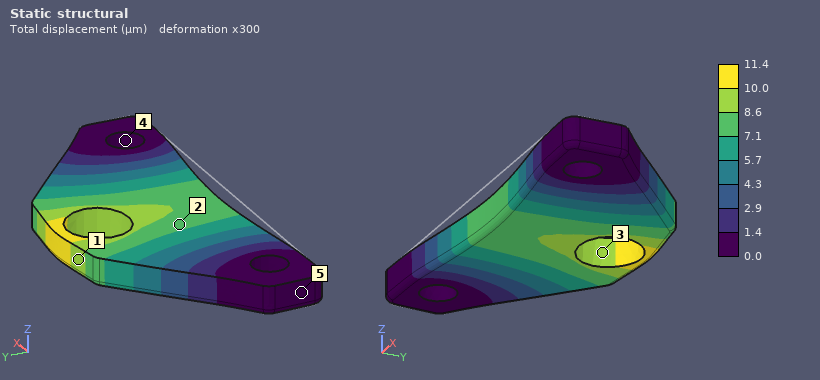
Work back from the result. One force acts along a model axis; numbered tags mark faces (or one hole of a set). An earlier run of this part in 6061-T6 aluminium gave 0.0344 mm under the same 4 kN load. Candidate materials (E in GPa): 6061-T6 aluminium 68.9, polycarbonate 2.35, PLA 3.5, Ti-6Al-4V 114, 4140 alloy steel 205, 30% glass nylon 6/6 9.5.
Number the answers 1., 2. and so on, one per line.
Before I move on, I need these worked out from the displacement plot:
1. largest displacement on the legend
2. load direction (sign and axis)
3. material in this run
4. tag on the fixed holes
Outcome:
1. 11.4 µm
2. +Y
3. 4140 alloy steel
4. 4
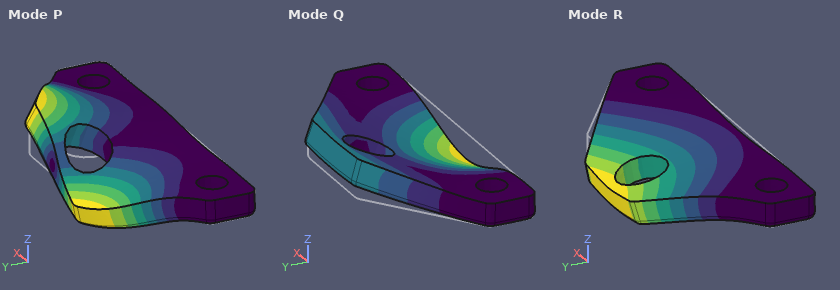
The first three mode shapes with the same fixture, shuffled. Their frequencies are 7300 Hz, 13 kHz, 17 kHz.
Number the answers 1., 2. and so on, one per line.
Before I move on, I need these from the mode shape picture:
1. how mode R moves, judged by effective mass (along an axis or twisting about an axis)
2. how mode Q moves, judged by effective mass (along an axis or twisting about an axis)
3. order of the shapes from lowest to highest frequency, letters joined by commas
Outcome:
1. along Z
2. along Z
3. R, Q, P
